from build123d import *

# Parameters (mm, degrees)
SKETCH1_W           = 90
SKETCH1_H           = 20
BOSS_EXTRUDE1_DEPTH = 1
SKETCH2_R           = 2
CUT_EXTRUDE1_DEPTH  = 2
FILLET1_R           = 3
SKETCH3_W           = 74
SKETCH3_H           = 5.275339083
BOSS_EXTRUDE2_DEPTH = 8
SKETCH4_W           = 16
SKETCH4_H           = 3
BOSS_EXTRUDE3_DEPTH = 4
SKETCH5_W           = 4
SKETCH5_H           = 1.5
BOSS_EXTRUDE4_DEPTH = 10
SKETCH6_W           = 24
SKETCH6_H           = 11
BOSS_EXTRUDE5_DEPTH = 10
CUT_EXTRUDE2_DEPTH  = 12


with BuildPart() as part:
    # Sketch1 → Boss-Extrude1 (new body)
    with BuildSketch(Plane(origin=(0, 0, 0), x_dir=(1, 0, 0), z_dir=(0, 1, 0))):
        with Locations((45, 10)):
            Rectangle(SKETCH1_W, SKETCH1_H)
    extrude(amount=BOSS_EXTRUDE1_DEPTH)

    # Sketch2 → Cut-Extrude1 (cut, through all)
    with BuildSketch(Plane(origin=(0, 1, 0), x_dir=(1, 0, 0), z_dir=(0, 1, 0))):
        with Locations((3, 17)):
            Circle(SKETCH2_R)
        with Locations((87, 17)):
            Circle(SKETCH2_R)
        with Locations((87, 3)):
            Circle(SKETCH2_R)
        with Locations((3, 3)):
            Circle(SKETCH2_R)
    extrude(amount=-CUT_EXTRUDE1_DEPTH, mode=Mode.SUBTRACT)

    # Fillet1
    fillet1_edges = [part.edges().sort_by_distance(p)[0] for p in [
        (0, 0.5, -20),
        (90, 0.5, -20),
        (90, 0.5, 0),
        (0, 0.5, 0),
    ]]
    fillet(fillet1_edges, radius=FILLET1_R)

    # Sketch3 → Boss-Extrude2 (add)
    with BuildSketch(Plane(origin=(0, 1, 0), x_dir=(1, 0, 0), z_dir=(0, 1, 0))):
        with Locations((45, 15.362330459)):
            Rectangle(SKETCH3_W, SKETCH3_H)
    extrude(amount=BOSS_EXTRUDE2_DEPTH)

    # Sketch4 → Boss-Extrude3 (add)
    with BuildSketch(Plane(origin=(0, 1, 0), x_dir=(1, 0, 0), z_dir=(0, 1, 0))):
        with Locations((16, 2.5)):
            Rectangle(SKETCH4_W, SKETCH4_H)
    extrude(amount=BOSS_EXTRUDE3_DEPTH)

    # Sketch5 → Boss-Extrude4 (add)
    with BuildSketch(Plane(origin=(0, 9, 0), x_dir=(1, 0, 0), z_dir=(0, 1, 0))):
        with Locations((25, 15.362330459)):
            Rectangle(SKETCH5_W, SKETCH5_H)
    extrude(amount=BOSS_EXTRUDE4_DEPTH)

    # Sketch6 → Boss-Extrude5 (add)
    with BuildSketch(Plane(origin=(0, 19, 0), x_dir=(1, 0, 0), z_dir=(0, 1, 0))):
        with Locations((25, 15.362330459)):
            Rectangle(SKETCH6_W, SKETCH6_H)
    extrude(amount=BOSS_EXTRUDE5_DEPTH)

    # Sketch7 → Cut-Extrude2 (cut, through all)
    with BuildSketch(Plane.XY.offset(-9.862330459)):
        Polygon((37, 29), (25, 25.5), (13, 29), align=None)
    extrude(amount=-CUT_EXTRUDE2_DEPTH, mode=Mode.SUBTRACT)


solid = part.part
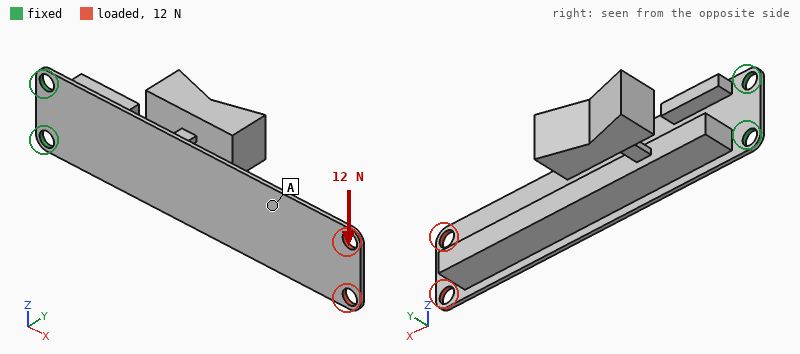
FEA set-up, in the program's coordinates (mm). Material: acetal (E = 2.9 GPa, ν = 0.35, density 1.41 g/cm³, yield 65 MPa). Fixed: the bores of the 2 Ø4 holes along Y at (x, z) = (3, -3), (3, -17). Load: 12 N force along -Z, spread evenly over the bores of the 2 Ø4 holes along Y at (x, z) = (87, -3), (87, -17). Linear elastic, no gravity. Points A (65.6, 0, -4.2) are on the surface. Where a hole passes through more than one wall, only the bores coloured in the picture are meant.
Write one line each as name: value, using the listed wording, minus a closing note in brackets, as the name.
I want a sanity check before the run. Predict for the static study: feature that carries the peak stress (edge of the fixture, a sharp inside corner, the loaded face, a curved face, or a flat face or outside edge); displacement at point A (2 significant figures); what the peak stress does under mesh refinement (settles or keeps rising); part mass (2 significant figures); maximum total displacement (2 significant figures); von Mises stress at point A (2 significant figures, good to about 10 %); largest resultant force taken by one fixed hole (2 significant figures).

feature that carries the peak stress: edge of the fixture
displacement at point A: 0.60 mm
what the peak stress does under mesh refinement: keeps rising
part mass: 10 g
maximum total displacement: 1.0 mm
von Mises stress at point A: 2.2 MPa
largest resultant force taken by one fixed hole: 67 N
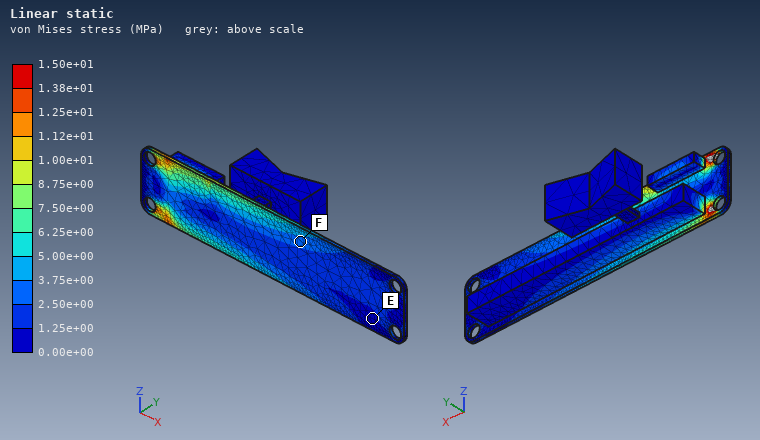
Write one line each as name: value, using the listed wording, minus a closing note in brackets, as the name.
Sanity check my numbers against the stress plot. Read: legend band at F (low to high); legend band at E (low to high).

legend band at F: 2.50e+00 to 3.75e+00 MPa
legend band at E: 0.00e+00 to 1.25e+00 MPa
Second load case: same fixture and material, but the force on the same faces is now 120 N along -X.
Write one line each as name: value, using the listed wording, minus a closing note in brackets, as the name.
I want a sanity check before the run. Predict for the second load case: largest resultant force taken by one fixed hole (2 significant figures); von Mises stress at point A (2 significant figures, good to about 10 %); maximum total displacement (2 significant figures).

largest resultant force taken by one fixed hole: 61 N
von Mises stress at point A: 6.0 MPa
maximum total displacement: 0.94 mm
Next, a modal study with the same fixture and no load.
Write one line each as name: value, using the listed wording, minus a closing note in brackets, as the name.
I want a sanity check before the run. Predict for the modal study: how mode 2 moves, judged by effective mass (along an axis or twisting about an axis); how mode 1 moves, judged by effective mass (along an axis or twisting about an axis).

how mode 2 moves, judged by effective mass: along Z
how mode 1 moves, judged by effective mass: along Y
